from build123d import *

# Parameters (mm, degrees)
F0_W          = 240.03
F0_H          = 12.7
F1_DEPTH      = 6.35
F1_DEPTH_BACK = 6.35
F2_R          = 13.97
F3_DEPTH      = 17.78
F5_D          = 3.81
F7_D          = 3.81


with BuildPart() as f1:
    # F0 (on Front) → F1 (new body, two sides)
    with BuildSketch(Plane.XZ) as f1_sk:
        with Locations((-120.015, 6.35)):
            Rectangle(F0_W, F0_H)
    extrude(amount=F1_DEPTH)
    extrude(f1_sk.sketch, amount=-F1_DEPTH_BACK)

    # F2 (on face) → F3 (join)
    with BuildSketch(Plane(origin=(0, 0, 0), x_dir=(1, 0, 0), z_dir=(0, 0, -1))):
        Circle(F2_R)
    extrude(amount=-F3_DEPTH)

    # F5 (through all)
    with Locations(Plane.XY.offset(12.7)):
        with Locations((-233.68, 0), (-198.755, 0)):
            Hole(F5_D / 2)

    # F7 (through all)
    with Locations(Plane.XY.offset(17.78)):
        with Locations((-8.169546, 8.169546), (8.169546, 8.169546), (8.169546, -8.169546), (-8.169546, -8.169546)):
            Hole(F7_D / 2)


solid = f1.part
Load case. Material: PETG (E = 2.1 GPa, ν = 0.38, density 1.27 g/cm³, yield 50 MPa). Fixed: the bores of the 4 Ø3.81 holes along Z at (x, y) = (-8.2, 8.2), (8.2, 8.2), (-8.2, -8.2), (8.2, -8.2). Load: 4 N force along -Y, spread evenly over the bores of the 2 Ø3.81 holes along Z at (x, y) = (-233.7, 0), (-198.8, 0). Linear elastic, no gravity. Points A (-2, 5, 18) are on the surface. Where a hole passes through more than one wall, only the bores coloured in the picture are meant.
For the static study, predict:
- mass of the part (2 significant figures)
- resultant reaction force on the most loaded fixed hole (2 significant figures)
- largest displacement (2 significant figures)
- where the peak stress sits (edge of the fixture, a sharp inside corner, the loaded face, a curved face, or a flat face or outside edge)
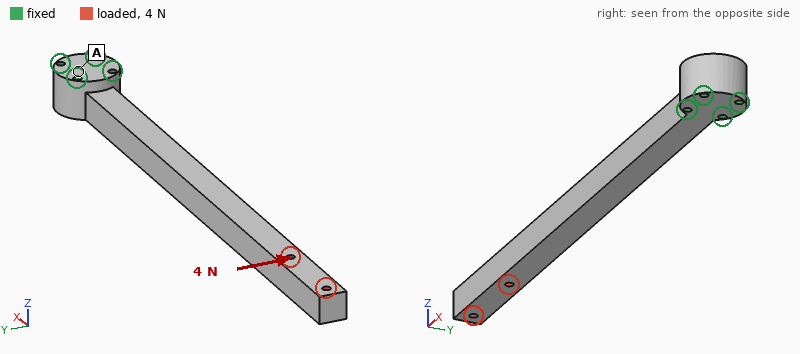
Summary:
59 g
53 N
3.0 mm
a flat face or outside edge
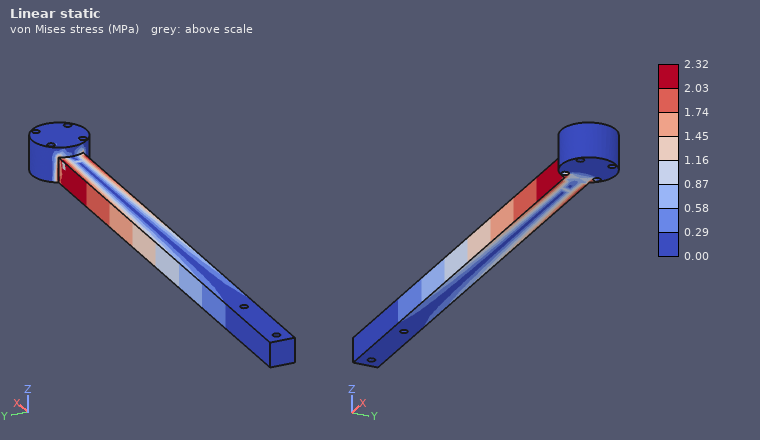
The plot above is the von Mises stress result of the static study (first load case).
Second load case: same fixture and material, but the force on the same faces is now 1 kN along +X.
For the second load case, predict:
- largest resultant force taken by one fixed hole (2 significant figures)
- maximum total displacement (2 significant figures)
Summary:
450 N
0.67 mm
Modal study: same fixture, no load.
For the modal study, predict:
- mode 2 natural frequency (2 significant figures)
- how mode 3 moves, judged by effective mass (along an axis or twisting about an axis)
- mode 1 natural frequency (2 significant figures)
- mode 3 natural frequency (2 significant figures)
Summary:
50 Hz
along Z
50 Hz
310 Hz
